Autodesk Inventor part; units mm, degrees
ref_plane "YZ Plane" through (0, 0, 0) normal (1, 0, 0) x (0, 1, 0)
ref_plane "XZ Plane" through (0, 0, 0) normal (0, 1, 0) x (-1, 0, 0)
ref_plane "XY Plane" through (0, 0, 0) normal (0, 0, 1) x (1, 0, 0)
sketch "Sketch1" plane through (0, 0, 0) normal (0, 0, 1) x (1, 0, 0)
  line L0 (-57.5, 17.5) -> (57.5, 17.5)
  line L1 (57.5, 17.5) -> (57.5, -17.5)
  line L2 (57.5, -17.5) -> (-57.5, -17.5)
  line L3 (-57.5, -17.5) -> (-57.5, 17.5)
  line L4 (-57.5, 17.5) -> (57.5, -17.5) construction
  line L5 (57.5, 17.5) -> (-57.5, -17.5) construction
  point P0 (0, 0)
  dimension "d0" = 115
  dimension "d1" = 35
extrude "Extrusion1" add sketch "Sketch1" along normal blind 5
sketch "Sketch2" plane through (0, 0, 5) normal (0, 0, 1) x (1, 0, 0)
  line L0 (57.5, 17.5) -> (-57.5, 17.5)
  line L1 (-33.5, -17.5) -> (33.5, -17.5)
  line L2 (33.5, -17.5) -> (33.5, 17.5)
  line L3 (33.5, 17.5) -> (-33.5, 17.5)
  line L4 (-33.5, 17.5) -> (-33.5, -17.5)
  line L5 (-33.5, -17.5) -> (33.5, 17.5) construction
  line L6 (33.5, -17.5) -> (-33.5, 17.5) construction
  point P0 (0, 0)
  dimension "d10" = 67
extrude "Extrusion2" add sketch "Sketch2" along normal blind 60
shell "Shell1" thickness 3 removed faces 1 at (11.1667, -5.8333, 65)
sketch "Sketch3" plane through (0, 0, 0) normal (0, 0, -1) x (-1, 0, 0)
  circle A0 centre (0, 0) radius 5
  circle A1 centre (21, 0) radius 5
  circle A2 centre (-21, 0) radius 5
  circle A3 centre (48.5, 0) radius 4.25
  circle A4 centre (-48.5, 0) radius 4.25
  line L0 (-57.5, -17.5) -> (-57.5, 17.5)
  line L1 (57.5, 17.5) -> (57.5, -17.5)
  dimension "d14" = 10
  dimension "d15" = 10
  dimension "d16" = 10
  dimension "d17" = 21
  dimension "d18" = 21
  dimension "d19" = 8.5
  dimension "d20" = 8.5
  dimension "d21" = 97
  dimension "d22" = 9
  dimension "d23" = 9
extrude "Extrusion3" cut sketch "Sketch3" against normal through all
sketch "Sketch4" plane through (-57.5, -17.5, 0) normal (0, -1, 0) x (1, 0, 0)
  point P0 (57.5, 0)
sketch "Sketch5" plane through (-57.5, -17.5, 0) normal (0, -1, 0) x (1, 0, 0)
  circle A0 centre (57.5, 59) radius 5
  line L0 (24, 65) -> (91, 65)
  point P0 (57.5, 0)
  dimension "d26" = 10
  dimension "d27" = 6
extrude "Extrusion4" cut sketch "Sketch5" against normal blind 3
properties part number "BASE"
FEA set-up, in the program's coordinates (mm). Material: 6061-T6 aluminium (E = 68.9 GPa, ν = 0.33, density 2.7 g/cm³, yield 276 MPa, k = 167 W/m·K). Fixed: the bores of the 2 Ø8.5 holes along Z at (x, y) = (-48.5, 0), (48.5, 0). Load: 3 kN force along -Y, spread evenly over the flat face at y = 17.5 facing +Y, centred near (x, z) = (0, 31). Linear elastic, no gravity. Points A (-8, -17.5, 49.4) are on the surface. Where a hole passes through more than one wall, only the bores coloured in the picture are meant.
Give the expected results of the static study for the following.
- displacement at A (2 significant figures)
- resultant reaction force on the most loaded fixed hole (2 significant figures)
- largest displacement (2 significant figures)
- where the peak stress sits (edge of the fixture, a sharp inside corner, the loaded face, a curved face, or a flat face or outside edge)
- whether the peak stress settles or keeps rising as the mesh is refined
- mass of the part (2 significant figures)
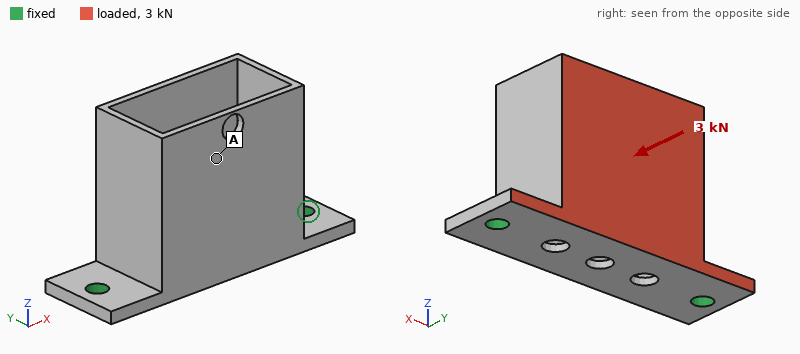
0.60 mm
1.5 kN
1.2 mm
edge of the fixture
keeps rising
130 g
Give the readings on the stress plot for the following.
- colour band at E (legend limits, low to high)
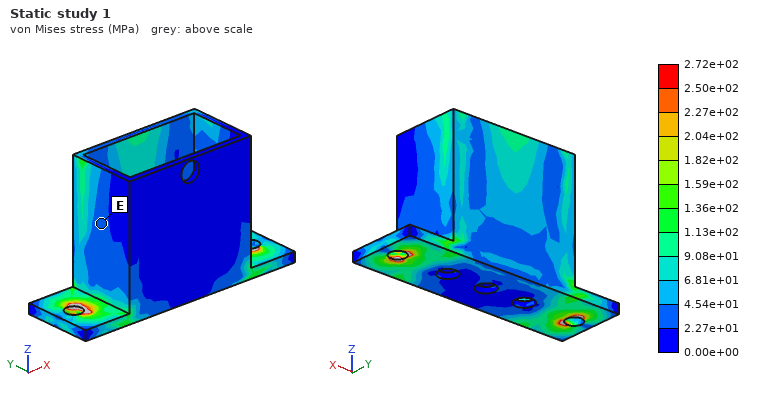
2.27e+01 to 4.54e+01 MPa
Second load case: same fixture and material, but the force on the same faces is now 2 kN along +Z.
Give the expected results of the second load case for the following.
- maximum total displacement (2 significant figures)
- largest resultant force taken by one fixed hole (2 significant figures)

0.35 mm
1.0 kN
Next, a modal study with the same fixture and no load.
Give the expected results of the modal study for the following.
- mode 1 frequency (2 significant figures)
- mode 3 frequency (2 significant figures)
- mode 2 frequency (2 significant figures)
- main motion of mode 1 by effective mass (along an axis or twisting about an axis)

1100 Hz
2900 Hz
2400 Hz
along Y
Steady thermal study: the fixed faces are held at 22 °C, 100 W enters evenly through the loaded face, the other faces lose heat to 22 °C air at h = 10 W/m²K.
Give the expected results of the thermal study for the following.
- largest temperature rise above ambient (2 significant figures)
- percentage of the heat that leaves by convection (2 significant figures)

80 K
11 %
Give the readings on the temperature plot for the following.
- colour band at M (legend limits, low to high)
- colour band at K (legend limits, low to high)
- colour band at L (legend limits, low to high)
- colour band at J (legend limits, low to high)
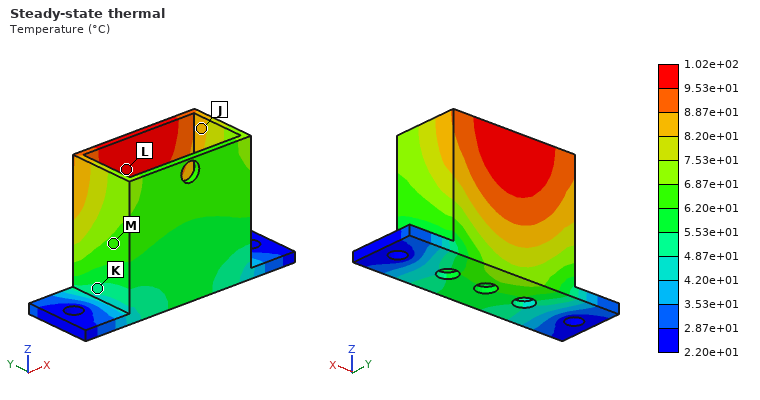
6.20e+01 to 6.87e+01 °C
4.87e+01 to 5.53e+01 °C
9.53e+01 to 1.02e+02 °C
8.20e+01 to 8.87e+01 °C
